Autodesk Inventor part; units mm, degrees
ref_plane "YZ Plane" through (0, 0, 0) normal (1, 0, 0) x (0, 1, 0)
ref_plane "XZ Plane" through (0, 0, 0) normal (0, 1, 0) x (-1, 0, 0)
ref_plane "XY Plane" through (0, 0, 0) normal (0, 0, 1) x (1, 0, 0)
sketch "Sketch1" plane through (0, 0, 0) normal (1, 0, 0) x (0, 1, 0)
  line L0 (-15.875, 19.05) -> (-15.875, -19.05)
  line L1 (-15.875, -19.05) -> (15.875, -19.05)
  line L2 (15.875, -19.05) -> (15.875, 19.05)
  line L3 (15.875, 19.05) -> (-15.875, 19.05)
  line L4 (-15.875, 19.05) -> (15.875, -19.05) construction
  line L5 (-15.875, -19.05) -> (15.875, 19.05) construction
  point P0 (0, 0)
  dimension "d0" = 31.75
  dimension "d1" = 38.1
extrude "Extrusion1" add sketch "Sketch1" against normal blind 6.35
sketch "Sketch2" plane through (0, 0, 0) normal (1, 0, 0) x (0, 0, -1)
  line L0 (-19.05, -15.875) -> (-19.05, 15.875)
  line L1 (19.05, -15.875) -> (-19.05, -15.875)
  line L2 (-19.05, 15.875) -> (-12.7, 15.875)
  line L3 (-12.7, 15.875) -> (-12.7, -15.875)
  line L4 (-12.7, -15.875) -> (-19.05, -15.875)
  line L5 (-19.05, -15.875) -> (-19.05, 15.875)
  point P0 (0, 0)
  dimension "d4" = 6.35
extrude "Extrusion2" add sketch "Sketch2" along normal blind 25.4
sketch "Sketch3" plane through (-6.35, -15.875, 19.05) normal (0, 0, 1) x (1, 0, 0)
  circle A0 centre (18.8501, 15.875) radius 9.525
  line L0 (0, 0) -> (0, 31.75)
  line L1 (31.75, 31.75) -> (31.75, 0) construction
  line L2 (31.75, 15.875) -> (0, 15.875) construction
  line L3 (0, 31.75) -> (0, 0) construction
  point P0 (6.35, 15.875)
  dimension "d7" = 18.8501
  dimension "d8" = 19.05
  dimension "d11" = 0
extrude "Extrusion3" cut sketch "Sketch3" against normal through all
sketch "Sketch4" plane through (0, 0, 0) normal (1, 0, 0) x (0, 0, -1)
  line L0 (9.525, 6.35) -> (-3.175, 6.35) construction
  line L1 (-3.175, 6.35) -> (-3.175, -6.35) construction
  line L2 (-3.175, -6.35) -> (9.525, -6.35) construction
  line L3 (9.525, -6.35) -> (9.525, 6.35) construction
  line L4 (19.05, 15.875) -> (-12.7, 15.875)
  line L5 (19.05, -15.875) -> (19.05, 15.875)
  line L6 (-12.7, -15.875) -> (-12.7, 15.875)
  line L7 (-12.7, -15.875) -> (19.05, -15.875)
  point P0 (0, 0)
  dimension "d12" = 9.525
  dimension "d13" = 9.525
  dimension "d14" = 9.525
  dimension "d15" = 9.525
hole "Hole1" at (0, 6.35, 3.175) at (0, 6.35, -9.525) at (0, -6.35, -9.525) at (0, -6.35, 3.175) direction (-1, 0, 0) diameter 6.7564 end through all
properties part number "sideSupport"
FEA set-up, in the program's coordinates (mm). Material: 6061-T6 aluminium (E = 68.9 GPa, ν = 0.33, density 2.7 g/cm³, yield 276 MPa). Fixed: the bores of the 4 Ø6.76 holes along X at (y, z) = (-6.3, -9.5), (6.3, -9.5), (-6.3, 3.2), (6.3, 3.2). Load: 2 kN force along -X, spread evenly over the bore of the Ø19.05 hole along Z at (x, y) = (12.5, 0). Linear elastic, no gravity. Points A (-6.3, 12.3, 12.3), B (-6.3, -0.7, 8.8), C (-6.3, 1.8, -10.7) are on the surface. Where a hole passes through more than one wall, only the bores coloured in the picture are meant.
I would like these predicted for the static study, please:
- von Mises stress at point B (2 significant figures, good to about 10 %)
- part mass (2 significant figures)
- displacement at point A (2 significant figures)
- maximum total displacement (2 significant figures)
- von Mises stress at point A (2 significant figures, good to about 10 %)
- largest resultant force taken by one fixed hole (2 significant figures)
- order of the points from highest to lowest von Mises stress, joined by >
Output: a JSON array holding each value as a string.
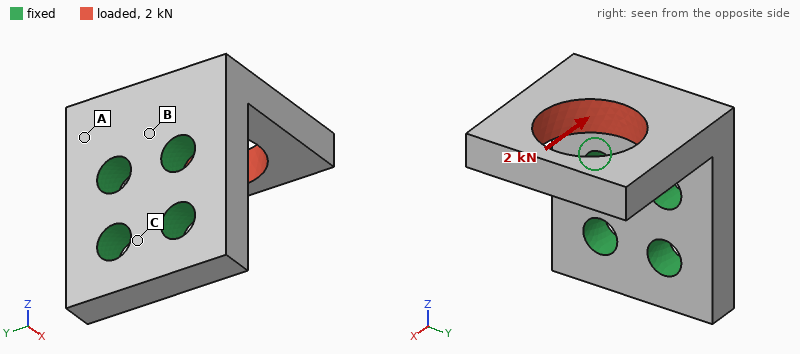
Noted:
["50 MPa", "27 g", "16 µm", "87 µm", "26 MPa", "1.1 kN", "B > A > C"]
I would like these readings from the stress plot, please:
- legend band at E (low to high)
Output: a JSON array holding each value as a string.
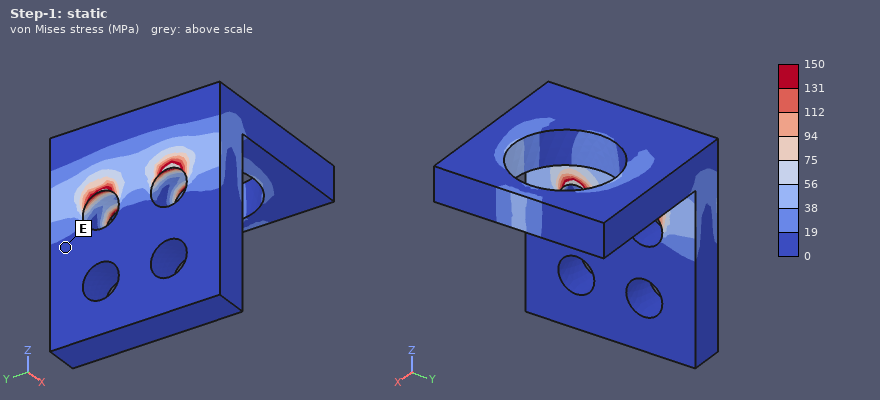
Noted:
["0 to 19 MPa"]
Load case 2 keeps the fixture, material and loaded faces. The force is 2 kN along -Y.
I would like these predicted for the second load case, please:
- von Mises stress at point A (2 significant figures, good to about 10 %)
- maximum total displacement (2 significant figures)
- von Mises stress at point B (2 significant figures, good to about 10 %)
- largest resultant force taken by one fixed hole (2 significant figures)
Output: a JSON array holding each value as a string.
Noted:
["37 MPa", "0.13 mm", "18 MPa", "2.1 kN"]
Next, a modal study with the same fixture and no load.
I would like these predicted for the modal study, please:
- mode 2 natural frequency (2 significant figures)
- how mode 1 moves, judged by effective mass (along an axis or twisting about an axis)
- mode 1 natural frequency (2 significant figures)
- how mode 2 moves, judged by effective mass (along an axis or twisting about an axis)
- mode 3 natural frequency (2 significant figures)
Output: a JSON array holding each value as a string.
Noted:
["7100 Hz", "along Z", "4300 Hz", "along Y", "9600 Hz"]
